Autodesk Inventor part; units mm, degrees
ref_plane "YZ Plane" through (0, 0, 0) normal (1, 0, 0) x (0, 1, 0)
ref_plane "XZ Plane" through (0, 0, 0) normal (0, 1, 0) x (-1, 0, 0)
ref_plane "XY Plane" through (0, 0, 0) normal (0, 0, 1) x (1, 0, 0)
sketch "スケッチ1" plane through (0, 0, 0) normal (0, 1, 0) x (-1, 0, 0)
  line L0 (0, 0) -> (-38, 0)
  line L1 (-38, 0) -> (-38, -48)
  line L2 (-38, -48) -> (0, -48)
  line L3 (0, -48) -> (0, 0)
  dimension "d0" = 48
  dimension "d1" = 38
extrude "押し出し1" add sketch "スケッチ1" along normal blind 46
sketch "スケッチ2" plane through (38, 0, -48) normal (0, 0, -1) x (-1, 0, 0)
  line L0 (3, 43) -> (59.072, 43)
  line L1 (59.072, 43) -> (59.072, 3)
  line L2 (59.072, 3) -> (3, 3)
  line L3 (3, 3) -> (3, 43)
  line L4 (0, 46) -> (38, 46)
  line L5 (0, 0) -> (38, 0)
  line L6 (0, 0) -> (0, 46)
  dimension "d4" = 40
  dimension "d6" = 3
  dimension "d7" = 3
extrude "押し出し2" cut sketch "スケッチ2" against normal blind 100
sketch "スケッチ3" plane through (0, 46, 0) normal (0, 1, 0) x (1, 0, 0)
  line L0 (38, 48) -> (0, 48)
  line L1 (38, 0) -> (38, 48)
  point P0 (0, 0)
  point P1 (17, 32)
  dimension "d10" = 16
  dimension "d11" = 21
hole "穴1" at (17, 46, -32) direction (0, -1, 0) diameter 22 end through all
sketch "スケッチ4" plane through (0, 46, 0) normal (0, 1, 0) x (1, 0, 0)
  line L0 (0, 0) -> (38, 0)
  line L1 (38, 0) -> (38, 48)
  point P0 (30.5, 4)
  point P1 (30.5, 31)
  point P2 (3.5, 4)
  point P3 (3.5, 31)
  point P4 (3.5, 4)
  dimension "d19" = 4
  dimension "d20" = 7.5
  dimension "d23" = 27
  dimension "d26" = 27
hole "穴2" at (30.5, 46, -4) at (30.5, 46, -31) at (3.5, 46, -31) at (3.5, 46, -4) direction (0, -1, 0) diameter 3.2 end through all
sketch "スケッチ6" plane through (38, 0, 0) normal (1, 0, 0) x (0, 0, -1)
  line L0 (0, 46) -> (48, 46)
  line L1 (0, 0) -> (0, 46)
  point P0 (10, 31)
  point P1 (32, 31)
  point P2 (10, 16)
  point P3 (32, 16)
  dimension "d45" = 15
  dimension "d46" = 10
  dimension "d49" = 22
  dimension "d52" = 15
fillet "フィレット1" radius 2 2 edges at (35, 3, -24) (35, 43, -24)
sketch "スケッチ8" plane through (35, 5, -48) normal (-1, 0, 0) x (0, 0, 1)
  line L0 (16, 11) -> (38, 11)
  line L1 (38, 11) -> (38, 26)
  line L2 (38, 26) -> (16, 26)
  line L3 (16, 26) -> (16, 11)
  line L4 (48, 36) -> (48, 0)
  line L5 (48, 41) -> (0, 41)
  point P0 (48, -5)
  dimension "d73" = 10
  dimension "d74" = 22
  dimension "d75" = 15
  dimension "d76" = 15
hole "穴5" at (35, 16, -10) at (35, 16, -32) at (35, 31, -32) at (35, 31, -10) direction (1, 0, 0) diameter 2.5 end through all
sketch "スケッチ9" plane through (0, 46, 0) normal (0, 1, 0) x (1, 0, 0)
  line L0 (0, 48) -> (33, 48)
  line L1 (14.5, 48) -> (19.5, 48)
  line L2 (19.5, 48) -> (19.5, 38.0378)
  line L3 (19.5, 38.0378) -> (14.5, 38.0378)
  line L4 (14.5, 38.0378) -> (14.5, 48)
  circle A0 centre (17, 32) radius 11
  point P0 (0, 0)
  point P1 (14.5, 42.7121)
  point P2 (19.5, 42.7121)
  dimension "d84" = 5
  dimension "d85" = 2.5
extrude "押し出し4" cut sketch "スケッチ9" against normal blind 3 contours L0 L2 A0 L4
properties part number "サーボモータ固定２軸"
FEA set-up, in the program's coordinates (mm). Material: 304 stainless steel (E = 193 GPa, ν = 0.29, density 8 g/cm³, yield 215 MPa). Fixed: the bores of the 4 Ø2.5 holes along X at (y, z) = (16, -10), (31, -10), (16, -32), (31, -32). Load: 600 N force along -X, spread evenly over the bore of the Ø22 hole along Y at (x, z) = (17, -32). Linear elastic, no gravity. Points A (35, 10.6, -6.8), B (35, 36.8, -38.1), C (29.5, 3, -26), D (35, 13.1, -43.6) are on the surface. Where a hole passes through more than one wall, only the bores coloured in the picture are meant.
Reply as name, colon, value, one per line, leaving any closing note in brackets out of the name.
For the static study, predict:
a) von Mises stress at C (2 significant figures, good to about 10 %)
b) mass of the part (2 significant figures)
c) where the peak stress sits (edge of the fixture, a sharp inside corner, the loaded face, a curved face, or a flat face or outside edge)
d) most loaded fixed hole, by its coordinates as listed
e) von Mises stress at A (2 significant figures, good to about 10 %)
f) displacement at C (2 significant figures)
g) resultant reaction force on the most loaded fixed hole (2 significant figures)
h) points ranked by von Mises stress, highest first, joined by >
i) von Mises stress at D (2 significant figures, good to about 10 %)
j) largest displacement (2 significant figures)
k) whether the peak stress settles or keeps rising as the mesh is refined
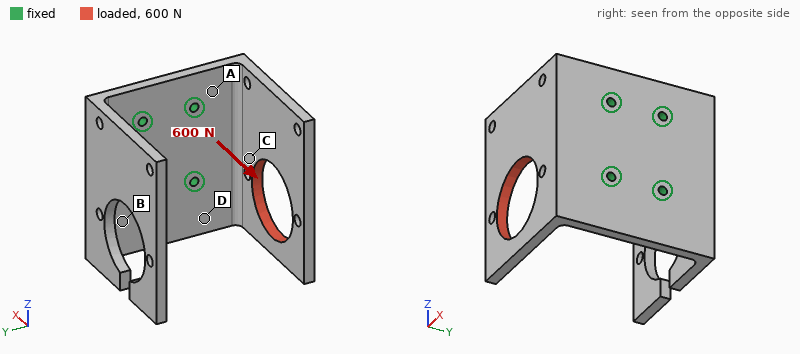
von Mises stress at C: 31 MPa
mass of the part: 110 g
where the peak stress sits: edge of the fixture
most loaded fixed hole, by its coordinates as listed: (16, -32)
von Mises stress at A: 61 MPa
displacement at C: 0.045 mm
resultant reaction force on the most loaded fixed hole: 710 N
points ranked by von Mises stress, highest first, joined by >: D > A > C > B
von Mises stress at D: 77 MPa
largest displacement: 0.16 mm
whether the peak stress settles or keeps rising as the mesh is refined: keeps rising
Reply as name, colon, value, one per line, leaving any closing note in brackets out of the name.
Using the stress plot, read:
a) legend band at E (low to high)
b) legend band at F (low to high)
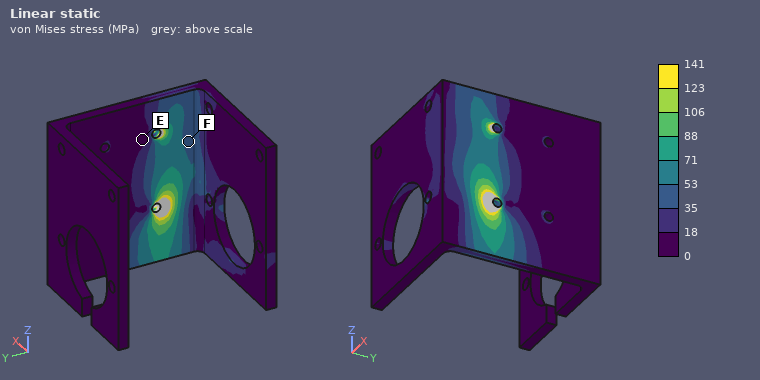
legend band at E: 0 to 18 MPa
legend band at F: 35 to 53 MPa
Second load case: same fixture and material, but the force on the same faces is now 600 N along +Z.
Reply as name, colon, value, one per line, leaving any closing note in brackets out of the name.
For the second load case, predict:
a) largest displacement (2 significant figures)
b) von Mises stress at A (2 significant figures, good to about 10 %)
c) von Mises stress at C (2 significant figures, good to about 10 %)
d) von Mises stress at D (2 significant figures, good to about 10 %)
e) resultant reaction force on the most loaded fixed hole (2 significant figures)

largest displacement: 98 µm
von Mises stress at A: 59 MPa
von Mises stress at C: 64 MPa
von Mises stress at D: 43 MPa
resultant reaction force on the most loaded fixed hole: 650 N
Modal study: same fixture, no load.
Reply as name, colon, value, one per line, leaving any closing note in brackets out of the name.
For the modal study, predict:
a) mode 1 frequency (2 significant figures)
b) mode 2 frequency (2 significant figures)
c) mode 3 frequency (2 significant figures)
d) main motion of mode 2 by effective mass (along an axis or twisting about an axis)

mode 1 frequency: 990 Hz
mode 2 frequency: 1200 Hz
mode 3 frequency: 1700 Hz
main motion of mode 2 by effective mass: along Y
